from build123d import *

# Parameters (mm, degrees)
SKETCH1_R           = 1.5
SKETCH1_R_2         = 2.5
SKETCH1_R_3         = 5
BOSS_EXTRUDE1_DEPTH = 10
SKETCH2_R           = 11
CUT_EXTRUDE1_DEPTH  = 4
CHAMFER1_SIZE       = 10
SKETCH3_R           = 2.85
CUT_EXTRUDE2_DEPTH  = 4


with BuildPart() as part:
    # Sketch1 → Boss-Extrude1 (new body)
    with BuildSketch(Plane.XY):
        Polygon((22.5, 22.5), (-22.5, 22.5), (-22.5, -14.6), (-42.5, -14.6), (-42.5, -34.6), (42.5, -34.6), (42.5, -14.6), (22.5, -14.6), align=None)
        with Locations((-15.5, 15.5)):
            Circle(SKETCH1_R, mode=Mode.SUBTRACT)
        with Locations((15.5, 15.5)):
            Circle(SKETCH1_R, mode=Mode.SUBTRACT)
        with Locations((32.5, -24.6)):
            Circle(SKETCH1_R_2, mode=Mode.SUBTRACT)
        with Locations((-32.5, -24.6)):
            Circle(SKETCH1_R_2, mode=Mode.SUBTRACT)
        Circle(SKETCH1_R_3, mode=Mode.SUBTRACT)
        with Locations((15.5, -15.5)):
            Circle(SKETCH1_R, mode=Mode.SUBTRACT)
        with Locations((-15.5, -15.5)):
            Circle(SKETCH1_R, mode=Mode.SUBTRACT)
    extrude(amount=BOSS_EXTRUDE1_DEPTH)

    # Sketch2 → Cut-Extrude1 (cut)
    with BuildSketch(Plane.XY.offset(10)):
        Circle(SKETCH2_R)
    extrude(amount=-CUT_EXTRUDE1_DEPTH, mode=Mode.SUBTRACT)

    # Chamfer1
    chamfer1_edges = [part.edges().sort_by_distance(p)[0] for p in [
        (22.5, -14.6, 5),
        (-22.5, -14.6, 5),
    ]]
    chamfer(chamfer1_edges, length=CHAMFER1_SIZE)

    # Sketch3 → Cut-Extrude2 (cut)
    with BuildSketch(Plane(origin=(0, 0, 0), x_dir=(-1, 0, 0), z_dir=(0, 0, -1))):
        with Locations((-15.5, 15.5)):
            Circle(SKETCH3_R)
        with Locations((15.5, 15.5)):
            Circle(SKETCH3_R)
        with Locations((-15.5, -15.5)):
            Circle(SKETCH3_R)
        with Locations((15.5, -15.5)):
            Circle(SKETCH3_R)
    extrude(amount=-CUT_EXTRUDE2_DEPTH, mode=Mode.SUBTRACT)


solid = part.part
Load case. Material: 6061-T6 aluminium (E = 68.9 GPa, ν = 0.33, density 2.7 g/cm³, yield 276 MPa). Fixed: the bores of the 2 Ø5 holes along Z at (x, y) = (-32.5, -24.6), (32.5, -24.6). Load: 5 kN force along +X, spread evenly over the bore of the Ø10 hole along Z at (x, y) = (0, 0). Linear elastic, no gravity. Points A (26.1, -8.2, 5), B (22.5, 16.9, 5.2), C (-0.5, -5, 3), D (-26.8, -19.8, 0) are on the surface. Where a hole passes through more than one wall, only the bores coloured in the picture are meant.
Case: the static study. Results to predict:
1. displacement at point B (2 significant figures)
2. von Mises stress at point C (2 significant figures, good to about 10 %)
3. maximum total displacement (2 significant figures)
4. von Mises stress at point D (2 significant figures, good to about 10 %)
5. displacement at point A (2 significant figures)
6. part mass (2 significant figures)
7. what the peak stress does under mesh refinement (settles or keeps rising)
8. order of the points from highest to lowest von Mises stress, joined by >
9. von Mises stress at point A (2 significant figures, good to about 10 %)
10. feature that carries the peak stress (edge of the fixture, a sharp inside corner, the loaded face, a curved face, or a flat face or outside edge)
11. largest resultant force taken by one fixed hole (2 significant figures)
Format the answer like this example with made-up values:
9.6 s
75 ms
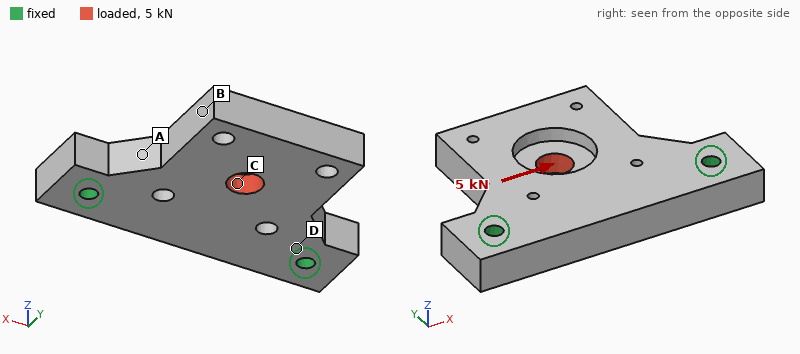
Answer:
19 µm
49 MPa
21 µm
19 MPa
7.2 µm
86 g
keeps rising
C > A > D > B
28 MPa
edge of the fixture
3.1 kN
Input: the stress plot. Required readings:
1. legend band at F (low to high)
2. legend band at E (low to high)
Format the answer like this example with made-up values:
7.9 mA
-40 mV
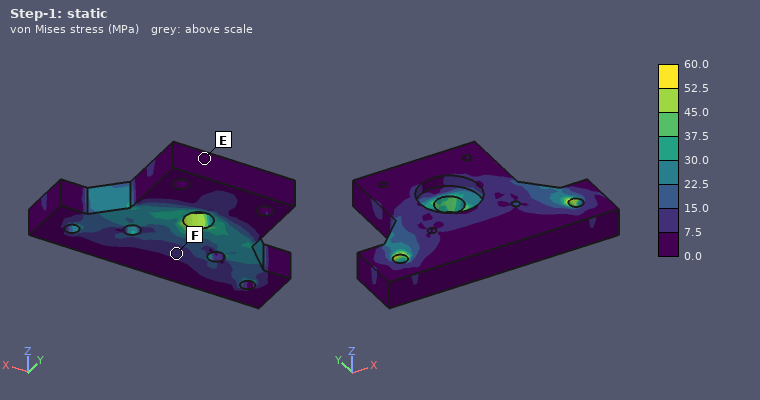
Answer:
7.5 to 15.0 MPa
0.0 to 7.5 MPa
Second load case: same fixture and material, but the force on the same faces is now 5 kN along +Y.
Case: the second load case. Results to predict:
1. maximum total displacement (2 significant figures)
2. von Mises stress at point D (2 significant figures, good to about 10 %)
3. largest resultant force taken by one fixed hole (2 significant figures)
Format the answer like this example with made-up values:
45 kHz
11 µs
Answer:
55 µm
40 MPa
2.8 kN
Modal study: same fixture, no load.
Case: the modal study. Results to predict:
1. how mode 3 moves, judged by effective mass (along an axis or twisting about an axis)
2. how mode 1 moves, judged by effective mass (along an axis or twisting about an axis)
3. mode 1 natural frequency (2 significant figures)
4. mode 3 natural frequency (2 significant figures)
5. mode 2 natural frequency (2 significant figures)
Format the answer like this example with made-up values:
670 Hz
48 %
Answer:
along Z
along Z
2800 Hz
10 kHz
7800 Hz
